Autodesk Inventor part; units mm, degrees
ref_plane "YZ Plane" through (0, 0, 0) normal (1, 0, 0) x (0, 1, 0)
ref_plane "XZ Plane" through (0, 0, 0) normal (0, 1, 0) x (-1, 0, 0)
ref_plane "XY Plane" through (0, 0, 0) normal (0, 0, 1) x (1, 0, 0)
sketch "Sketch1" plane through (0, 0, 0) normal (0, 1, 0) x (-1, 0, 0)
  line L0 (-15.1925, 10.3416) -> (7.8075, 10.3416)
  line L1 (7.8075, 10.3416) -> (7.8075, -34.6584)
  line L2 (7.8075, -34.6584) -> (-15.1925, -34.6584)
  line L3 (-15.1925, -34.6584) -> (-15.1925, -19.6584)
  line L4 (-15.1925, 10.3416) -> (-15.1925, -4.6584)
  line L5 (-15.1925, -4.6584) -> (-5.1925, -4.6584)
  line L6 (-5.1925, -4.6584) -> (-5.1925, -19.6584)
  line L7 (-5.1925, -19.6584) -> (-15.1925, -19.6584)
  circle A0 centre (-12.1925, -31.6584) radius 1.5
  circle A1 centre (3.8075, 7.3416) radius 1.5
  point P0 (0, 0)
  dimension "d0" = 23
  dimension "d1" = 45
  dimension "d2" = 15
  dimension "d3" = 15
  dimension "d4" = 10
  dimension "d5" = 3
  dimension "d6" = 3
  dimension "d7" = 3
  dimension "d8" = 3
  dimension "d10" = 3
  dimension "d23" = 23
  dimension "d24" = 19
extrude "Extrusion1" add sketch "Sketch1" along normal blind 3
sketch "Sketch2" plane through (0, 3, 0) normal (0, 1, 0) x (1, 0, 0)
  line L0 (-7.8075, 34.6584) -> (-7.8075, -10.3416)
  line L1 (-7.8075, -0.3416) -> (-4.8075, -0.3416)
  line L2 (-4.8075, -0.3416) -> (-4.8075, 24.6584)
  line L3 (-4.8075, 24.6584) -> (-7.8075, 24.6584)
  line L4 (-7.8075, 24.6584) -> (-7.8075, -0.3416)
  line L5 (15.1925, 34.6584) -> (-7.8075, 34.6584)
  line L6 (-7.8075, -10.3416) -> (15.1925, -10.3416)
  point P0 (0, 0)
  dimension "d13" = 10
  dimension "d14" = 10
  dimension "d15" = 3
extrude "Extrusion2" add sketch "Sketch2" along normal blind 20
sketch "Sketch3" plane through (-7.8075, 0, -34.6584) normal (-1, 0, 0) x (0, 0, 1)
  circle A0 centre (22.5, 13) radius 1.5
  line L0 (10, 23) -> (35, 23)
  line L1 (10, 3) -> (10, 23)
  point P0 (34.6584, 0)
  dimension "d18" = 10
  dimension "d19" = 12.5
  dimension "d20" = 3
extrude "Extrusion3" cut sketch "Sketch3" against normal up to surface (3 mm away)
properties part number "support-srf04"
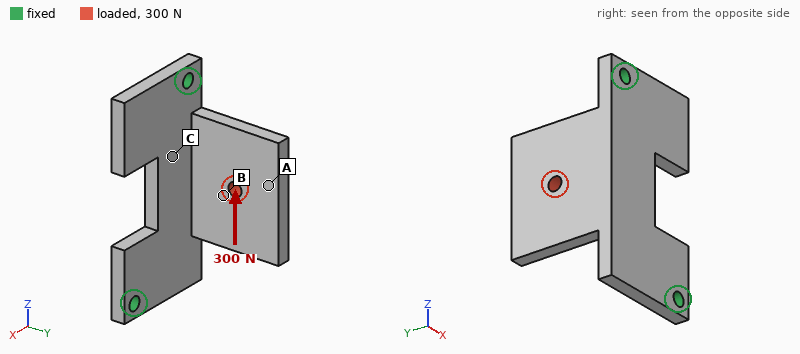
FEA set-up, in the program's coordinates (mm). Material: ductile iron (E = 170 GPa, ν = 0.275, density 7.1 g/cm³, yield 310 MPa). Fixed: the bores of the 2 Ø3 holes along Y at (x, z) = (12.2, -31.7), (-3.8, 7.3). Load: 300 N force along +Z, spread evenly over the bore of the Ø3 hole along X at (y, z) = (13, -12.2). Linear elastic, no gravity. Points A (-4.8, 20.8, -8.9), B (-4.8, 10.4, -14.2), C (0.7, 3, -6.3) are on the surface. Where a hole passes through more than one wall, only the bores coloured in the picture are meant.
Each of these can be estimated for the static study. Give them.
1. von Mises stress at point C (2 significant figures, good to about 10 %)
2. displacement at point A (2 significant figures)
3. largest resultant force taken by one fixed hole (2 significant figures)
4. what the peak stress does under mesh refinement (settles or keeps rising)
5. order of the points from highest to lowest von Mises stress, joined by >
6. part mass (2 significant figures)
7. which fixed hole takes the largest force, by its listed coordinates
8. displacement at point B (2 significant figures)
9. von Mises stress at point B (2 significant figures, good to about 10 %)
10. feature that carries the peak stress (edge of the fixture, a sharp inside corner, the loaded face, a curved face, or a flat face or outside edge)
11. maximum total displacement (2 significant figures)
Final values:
24 MPa
30 µm
270 N
keeps rising
C > B > A
29 g
(-3.8, 7.3)
21 µm
14 MPa
edge of the fixture
46 µm
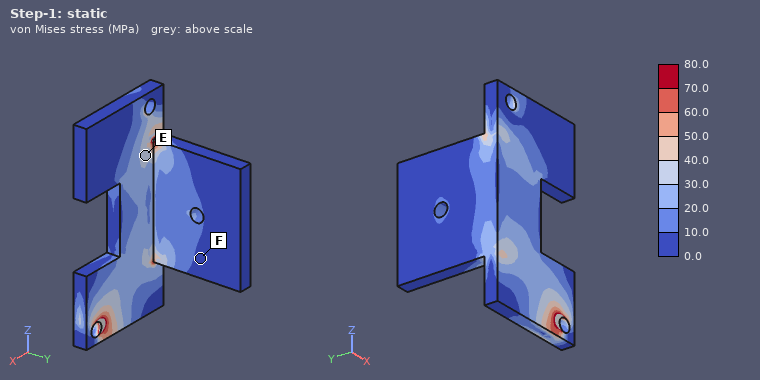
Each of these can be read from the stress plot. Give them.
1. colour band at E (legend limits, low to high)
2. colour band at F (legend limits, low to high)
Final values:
30.0 to 40.0 MPa
0.0 to 10.0 MPa
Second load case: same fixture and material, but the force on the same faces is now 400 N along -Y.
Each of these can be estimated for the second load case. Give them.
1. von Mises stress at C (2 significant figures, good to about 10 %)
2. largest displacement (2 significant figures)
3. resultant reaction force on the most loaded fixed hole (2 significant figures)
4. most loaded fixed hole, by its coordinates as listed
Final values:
31 MPa
89 µm
240 N
(-3.8, 7.3)
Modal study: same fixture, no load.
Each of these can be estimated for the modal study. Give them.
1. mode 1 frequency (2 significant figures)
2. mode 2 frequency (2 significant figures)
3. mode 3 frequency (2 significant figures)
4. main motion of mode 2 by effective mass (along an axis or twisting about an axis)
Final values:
2600 Hz
4500 Hz
6900 Hz
along Y
